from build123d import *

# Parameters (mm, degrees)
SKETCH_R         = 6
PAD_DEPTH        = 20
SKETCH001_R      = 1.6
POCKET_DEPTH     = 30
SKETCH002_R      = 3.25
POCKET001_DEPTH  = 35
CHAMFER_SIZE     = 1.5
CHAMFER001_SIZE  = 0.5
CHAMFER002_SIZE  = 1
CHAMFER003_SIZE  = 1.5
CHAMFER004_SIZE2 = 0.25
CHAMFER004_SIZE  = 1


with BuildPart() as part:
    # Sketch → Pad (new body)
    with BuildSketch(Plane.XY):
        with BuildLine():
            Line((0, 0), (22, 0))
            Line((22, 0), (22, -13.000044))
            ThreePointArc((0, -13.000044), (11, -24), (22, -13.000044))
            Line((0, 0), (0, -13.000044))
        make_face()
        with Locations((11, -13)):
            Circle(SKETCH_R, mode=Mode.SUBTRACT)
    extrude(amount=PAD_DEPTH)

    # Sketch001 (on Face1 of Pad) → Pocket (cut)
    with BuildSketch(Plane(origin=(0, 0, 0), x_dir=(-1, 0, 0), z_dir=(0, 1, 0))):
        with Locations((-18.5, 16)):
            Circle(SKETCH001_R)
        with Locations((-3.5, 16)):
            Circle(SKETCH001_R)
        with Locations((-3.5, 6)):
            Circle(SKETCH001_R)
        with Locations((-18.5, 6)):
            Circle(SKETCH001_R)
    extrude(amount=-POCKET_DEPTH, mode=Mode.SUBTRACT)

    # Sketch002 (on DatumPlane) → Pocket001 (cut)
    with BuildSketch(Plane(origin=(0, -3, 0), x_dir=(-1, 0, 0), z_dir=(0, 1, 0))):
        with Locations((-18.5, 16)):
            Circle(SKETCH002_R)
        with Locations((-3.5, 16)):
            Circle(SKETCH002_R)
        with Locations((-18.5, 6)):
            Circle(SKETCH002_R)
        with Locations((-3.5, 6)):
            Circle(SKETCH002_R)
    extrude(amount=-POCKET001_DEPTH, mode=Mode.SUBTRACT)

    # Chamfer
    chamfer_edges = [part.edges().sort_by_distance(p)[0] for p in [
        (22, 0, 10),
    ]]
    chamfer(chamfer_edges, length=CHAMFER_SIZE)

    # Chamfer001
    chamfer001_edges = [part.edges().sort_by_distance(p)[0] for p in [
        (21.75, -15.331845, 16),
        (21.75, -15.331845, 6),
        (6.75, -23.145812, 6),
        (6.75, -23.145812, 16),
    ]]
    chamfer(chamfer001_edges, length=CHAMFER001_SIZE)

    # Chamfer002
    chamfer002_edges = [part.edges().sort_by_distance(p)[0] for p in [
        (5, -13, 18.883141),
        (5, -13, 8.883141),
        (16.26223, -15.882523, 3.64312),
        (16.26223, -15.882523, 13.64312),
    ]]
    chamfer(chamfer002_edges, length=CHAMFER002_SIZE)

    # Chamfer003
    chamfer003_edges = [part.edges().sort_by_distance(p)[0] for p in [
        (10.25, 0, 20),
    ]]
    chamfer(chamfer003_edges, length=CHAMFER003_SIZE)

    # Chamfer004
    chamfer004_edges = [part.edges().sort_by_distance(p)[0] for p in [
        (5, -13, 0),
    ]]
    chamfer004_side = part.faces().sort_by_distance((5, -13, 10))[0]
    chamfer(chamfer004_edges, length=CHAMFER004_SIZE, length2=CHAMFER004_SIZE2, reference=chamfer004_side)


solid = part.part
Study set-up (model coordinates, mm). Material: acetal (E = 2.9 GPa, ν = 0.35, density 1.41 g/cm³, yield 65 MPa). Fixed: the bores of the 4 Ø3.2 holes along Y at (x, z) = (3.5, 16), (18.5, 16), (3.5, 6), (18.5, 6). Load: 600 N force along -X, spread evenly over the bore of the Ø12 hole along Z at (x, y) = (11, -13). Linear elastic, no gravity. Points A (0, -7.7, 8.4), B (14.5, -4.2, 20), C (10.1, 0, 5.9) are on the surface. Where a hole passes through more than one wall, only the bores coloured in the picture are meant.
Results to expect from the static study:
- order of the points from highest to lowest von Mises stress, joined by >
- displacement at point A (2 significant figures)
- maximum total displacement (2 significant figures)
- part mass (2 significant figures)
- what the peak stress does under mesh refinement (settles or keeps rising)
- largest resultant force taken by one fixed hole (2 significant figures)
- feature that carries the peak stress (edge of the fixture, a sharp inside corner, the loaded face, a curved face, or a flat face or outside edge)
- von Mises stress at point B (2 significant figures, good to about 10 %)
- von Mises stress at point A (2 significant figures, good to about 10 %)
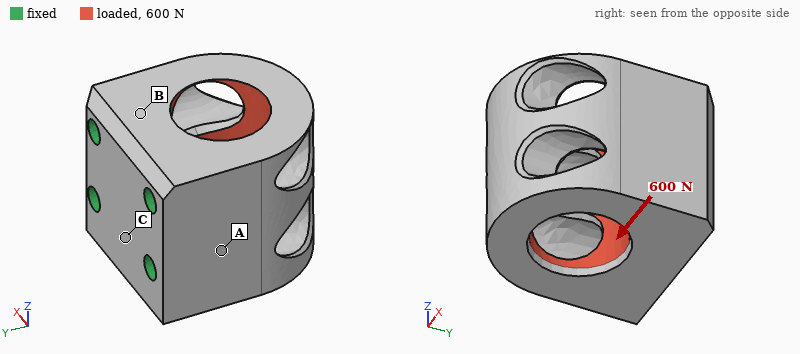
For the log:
A > B > C
0.061 mm
0.22 mm
6.8 g
keeps rising
280 N
edge of the fixture
6.7 MPa
12 MPa
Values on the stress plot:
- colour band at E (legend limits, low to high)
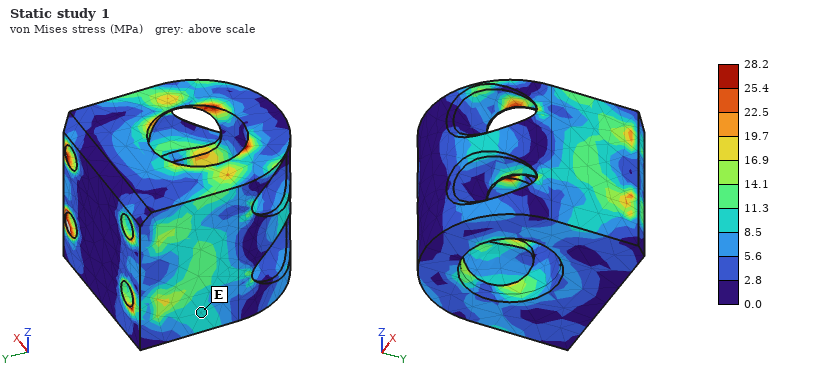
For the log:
8.5 to 11.3 MPa
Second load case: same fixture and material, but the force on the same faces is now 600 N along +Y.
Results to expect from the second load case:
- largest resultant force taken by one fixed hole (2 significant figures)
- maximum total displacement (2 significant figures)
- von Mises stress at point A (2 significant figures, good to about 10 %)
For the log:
170 N
72 µm
4.8 MPa
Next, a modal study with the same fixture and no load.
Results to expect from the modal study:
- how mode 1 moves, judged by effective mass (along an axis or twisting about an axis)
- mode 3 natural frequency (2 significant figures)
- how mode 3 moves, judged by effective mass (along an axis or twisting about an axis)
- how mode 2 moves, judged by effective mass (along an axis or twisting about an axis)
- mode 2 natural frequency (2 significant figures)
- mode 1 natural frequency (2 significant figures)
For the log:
along Z
6400 Hz
twisting about Y
along X
4300 Hz
3200 Hz
